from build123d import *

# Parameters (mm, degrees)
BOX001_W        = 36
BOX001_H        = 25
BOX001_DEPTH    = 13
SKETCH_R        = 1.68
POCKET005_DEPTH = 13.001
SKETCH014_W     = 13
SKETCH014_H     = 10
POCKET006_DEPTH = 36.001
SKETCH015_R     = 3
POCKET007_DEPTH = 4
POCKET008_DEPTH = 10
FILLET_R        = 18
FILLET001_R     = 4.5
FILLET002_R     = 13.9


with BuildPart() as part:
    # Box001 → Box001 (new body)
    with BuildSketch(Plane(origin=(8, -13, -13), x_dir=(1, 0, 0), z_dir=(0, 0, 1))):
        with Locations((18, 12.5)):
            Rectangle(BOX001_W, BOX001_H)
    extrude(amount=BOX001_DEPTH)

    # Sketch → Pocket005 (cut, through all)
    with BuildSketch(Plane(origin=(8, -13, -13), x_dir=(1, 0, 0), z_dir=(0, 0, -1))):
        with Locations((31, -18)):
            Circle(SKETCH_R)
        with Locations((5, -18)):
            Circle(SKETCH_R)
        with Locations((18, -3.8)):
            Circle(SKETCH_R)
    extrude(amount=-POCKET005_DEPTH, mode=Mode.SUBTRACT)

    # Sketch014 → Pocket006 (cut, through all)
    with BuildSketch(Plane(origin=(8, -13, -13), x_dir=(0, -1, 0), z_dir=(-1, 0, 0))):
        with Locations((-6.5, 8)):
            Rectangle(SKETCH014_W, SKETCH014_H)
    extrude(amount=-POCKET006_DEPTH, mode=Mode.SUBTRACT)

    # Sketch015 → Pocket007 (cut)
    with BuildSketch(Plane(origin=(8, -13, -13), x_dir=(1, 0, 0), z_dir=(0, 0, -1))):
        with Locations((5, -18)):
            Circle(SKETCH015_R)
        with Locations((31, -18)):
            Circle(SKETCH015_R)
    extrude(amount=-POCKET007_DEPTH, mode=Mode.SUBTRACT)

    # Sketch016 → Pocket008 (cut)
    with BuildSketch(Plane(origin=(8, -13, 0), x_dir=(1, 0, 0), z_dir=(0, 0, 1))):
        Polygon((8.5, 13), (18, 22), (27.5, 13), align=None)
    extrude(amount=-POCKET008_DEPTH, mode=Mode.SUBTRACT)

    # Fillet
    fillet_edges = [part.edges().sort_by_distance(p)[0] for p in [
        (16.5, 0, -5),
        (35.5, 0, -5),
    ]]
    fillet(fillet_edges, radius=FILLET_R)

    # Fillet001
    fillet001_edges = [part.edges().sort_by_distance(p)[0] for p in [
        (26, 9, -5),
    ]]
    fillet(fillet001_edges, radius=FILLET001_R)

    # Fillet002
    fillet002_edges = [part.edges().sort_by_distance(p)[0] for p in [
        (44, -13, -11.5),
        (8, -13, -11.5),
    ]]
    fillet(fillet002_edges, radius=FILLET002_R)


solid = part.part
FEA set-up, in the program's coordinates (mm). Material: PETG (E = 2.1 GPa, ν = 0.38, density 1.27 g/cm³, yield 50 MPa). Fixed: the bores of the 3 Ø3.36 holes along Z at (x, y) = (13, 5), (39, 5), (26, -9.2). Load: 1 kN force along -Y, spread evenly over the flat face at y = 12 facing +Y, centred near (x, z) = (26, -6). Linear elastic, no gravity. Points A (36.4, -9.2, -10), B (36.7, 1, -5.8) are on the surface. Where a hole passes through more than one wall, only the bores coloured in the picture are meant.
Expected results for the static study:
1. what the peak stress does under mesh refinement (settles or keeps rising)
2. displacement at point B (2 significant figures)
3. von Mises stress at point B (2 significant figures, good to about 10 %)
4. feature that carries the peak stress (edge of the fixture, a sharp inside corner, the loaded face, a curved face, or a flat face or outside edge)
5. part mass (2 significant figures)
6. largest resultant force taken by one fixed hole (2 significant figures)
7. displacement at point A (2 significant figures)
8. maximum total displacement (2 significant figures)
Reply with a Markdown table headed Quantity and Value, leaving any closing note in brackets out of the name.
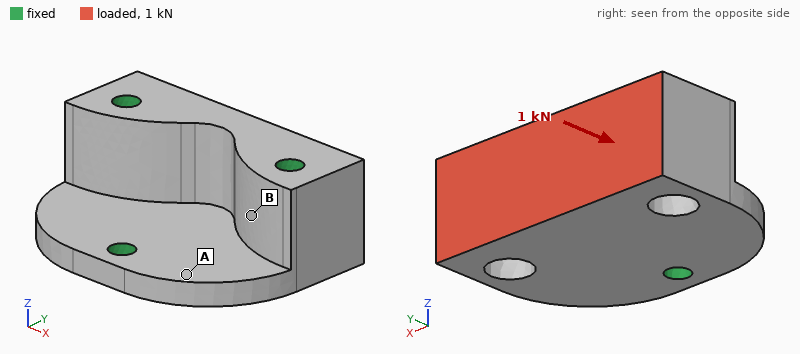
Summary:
| Quantity | Value |
|---|---|
| what the peak stress does under mesh refinement | keeps rising |
| displacement at point B | 11 µm |
| von Mises stress at point B | 4.1 MPa |
| feature that carries the peak stress | edge of the fixture |
| part mass | 6.9 g |
| largest resultant force taken by one fixed hole | 450 N |
| displacement at point A | 18 µm |
| maximum total displacement | 46 µm |
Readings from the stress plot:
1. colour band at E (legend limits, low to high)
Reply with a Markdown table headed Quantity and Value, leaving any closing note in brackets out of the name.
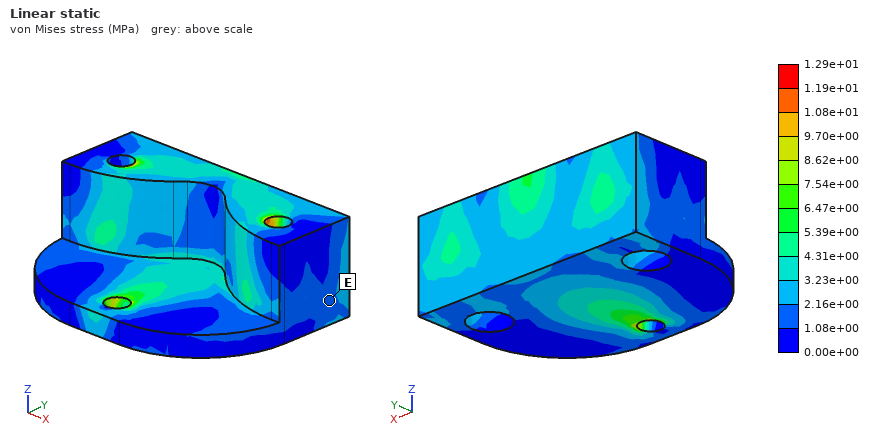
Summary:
| Quantity | Value |
|---|---|
| colour band at E | 1.08e+00 to 2.16e+00 MPa |
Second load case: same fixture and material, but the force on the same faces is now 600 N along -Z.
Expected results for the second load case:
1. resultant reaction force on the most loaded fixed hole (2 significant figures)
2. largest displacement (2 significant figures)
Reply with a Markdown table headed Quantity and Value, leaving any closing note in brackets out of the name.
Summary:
| Quantity | Value |
|---|---|
| resultant reaction force on the most loaded fixed hole | 320 N |
| largest displacement | 84 µm |
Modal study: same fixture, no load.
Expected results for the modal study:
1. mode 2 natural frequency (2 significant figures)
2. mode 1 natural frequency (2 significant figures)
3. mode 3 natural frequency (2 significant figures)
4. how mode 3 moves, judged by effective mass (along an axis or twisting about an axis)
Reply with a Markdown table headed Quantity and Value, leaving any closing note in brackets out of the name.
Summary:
| Quantity | Value |
|---|---|
| mode 2 natural frequency | 7200 Hz |
| mode 1 natural frequency | 7200 Hz |
| mode 3 natural frequency | 10 kHz |
| how mode 3 moves, judged by effective mass | along Z |
